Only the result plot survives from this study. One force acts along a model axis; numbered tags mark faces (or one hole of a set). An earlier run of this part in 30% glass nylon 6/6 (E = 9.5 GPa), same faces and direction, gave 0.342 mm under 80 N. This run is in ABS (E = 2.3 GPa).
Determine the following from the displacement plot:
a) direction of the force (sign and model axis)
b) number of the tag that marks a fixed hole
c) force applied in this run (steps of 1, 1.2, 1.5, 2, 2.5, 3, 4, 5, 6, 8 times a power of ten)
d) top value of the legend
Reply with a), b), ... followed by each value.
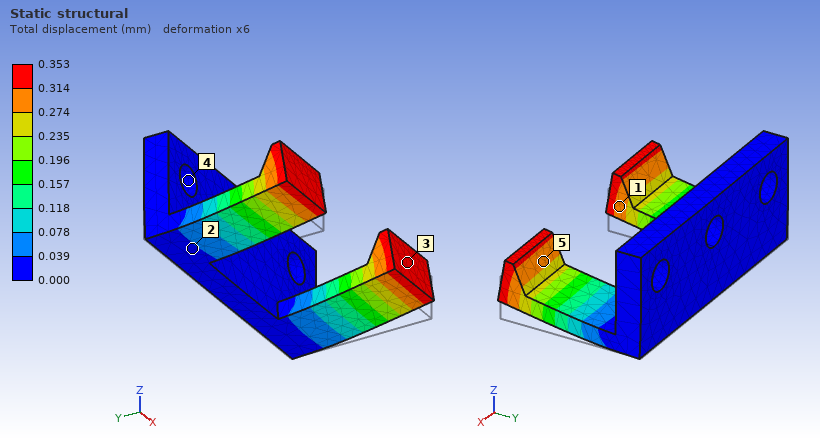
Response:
a) +Z
b) 4
c) 20 N
d) 0.353 mm
